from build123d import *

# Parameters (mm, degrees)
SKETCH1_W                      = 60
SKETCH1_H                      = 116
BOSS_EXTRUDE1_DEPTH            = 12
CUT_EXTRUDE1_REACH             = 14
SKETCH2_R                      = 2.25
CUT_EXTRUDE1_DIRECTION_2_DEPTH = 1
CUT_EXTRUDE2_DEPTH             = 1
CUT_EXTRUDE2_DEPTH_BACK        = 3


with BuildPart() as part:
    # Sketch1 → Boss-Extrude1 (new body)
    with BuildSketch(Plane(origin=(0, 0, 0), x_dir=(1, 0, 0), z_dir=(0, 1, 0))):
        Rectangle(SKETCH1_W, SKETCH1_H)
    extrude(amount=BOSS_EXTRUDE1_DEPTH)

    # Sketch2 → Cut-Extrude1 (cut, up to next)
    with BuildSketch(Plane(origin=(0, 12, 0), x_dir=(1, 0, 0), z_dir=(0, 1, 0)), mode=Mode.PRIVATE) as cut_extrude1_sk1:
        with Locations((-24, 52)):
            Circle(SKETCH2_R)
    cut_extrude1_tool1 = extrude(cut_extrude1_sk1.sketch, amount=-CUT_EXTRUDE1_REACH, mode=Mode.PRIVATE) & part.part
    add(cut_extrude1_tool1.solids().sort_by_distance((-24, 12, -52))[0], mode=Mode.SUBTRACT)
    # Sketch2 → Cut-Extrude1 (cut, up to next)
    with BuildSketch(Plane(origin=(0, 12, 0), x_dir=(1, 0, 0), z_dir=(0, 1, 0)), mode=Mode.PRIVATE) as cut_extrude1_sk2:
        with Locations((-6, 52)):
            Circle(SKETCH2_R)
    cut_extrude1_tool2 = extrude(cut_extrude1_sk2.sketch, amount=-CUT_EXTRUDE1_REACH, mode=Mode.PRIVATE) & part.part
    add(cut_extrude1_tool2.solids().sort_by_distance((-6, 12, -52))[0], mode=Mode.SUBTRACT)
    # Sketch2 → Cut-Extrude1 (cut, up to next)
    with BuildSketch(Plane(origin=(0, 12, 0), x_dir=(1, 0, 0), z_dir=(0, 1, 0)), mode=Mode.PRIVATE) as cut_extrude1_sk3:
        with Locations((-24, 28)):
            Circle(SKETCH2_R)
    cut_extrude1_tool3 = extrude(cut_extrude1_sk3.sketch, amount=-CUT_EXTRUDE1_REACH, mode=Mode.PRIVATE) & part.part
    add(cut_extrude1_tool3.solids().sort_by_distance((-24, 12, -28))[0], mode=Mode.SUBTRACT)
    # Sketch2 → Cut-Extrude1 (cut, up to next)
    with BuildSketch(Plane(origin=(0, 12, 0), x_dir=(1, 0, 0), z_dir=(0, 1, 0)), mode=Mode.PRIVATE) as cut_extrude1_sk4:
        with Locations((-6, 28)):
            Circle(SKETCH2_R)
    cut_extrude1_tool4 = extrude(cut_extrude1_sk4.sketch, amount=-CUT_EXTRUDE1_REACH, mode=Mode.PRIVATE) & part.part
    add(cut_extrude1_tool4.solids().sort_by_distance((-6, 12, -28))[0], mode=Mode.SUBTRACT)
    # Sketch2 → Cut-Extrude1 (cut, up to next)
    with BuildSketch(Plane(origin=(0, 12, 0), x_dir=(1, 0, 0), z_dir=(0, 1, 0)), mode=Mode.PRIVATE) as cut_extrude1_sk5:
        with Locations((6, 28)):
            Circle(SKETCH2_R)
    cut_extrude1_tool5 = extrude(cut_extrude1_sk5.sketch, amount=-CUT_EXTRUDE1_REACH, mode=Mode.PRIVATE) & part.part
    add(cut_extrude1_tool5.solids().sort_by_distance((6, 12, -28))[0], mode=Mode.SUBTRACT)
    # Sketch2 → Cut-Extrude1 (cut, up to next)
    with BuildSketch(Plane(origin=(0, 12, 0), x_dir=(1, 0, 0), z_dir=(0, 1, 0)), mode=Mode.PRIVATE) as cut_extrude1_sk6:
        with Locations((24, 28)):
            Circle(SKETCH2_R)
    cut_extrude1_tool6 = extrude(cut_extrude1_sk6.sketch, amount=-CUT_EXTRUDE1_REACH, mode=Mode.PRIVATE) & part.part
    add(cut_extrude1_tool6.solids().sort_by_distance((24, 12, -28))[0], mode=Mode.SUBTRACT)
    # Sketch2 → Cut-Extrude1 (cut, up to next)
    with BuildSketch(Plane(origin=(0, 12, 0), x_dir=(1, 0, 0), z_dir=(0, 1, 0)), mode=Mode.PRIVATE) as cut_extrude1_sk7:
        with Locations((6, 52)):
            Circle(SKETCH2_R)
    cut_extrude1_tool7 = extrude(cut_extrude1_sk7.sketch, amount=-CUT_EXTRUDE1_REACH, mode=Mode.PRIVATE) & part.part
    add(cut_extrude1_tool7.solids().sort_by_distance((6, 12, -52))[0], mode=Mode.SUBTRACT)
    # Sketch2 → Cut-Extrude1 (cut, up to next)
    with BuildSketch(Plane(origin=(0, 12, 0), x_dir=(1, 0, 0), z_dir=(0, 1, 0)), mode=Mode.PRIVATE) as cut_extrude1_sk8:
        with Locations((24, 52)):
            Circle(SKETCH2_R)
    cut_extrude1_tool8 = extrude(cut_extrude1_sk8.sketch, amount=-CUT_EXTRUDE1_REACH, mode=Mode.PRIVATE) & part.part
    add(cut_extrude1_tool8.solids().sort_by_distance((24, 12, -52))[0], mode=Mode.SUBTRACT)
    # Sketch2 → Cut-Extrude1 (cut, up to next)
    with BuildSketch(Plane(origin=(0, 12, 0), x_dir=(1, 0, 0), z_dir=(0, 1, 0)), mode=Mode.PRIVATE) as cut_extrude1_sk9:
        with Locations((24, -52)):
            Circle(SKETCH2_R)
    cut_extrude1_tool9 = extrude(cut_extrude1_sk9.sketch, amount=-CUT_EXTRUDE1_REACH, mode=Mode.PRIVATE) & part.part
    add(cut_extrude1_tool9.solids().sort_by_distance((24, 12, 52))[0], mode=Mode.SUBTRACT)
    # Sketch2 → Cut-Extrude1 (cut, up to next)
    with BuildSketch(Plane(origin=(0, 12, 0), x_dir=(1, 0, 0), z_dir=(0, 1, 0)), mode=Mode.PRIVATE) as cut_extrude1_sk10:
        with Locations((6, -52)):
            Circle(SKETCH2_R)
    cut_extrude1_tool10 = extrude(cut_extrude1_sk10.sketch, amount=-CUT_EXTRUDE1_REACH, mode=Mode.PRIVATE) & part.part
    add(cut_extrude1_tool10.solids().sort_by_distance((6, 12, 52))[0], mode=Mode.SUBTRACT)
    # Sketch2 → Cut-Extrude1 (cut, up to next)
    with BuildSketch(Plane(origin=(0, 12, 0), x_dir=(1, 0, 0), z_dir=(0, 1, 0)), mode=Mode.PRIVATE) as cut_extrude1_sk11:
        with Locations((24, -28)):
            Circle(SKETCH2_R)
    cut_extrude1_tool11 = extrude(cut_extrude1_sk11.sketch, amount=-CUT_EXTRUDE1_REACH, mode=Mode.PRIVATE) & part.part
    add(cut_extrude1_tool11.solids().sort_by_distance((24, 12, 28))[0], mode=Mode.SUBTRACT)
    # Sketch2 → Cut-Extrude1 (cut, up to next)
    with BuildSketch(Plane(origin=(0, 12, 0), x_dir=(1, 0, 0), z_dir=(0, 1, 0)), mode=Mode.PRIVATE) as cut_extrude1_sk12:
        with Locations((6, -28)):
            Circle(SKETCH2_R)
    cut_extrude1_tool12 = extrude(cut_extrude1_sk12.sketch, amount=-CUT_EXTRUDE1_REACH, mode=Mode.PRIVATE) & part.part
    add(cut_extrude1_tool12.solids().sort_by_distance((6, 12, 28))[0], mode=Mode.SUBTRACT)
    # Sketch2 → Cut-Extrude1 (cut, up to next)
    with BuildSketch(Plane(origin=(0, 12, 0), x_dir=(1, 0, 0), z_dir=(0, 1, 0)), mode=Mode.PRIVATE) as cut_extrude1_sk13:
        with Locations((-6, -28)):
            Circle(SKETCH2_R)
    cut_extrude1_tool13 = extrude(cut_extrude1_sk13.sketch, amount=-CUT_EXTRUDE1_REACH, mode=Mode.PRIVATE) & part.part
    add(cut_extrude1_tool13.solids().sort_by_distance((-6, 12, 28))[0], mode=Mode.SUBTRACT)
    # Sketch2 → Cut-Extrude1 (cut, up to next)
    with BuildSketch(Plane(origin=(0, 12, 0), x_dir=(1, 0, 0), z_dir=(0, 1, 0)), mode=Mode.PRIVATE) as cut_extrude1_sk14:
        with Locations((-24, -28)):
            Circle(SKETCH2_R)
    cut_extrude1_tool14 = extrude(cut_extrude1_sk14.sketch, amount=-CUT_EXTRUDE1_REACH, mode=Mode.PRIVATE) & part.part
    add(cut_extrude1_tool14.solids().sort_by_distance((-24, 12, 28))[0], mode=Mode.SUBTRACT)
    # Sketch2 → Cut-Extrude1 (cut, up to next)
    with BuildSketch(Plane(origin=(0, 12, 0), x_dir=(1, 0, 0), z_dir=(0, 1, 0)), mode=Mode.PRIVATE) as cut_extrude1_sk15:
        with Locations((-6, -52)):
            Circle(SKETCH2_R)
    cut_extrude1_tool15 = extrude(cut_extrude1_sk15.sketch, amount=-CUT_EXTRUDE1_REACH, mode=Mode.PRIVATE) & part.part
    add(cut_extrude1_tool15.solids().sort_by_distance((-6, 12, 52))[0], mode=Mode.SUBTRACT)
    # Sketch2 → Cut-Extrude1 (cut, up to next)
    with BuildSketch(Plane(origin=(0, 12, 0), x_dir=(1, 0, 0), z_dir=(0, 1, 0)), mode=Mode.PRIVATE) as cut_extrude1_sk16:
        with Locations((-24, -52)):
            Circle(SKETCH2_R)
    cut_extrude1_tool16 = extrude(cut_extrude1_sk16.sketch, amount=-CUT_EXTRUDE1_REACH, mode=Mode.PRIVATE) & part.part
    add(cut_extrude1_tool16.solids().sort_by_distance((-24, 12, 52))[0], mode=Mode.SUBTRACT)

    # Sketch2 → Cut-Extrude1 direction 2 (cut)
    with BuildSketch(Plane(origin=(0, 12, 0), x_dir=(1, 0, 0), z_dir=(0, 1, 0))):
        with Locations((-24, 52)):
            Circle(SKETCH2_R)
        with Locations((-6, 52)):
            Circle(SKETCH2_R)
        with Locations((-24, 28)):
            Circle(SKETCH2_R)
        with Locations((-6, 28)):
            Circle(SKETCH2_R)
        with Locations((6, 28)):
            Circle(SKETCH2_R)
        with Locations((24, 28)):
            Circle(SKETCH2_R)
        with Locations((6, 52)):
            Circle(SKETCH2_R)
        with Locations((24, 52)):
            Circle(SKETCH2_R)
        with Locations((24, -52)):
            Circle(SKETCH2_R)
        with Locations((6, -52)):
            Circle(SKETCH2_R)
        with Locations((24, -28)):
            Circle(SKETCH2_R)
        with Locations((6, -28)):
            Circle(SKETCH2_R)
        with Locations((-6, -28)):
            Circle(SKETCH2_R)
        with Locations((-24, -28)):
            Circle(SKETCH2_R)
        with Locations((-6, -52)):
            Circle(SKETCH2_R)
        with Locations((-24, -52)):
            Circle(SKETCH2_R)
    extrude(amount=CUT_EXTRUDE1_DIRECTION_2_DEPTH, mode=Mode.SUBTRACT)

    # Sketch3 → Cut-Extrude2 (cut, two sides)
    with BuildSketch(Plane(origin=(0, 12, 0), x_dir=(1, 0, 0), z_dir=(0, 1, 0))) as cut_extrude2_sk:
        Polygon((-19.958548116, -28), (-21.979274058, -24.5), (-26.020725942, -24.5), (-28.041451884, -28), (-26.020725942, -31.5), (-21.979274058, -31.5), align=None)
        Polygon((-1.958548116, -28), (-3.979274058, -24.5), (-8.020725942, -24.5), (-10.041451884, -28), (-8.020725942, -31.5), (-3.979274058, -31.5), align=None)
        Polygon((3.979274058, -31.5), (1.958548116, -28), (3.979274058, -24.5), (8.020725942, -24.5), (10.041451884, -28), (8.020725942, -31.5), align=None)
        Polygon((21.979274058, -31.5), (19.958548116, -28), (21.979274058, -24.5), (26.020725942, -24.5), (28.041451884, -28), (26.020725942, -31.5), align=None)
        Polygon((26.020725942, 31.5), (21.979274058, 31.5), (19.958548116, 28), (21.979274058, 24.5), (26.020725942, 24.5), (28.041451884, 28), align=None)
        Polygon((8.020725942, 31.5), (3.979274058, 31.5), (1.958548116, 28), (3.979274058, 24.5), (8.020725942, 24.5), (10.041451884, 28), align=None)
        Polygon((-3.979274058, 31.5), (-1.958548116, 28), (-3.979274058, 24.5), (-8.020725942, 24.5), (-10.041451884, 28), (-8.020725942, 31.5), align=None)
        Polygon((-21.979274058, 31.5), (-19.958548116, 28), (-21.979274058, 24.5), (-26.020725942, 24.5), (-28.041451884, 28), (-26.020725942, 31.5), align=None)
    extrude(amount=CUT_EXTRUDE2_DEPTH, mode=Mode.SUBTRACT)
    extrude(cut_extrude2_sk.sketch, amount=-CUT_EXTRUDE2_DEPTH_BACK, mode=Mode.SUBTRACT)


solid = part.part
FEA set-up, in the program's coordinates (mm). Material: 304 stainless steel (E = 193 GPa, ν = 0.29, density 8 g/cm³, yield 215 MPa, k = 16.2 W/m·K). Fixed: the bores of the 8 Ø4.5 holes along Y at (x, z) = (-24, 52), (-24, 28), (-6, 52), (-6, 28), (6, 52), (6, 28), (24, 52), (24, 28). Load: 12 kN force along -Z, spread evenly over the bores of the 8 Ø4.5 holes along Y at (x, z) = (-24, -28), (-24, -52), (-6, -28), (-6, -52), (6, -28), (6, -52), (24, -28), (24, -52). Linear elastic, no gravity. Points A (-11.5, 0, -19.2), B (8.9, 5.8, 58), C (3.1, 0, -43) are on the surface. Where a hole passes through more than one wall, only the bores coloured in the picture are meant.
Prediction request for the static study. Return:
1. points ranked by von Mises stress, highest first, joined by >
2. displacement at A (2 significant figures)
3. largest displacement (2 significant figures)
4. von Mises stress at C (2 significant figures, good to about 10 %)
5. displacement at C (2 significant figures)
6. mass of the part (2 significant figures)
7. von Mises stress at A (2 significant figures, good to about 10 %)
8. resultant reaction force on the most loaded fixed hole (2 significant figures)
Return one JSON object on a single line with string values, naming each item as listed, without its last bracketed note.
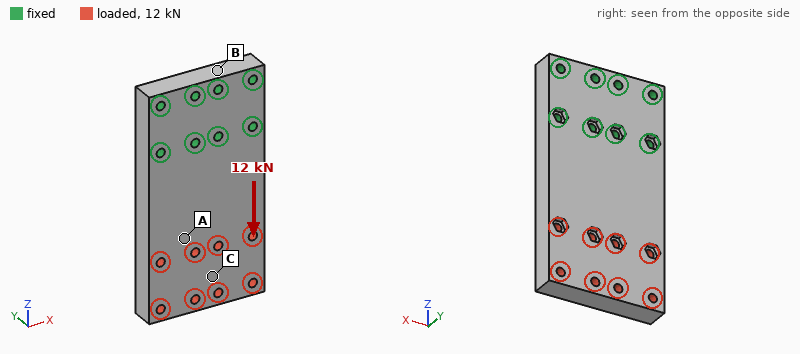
{"points ranked by von Mises stress, highest first, joined by >": "A > C > B", "displacement at A": "6.0 µm", "largest displacement": "12 µm", "von Mises stress at C": "11 MPa", "displacement at C": "10 µm", "mass of the part": "640 g", "von Mises stress at A": "22 MPa", "resultant reaction force on the most loaded fixed hole": "2.9 kN"}
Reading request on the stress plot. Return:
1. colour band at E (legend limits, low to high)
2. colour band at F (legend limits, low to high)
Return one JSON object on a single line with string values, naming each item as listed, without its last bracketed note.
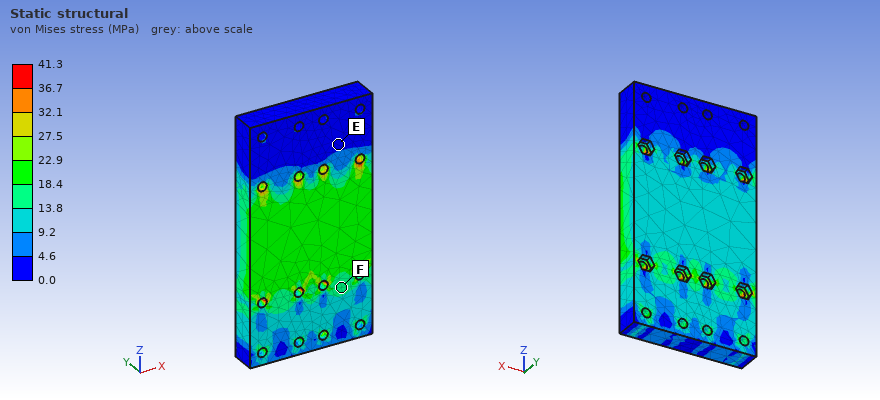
{"colour band at E": "0.0 to 4.6 MPa", "colour band at F": "13.8 to 18.4 MPa"}
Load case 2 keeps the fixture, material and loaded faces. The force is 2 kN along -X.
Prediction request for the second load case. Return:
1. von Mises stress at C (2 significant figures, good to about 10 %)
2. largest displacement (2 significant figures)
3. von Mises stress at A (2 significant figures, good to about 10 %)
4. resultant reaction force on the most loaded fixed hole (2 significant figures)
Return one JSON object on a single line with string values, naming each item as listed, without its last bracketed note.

{"von Mises stress at C": "4.7 MPa", "largest displacement": "12 µm", "von Mises stress at A": "6.7 MPa", "resultant reaction force on the most loaded fixed hole": "2.4 kN"}
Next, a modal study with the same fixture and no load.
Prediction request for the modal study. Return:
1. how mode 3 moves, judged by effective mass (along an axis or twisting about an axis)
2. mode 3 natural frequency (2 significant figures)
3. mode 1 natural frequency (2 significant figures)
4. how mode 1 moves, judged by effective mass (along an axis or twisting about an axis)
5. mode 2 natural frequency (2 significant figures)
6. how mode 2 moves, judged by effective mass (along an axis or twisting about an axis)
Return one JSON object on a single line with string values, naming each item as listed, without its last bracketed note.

{"how mode 3 moves, judged by effective mass": "along X", "mode 3 natural frequency": "4900 Hz", "mode 1 natural frequency": "1200 Hz", "how mode 1 moves, judged by effective mass": "along Y", "mode 2 natural frequency": "3700 Hz", "how mode 2 moves, judged by effective mass": "twisting about Z"}
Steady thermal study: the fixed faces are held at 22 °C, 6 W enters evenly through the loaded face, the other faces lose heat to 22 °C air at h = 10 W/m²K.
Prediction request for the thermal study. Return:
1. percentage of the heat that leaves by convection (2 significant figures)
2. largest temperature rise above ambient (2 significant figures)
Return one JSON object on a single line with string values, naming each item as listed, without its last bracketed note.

{"percentage of the heat that leaves by convection": "34 %", "largest temperature rise above ambient": "28 K"}
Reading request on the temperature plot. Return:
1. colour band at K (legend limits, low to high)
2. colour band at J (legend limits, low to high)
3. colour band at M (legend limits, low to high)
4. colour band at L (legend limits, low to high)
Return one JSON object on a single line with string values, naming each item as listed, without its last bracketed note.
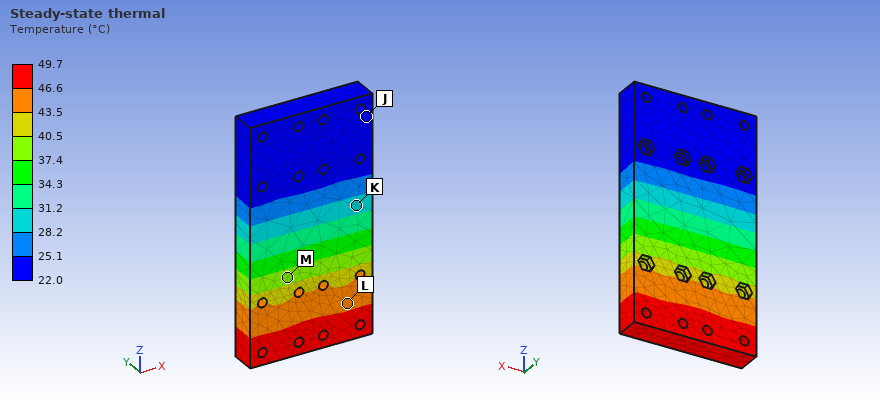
{"colour band at K": "28.2 to 31.2 °C", "colour band at J": "22.0 to 25.1 °C", "colour band at M": "37.4 to 40.5 °C", "colour band at L": "43.5 to 46.6 °C"}
